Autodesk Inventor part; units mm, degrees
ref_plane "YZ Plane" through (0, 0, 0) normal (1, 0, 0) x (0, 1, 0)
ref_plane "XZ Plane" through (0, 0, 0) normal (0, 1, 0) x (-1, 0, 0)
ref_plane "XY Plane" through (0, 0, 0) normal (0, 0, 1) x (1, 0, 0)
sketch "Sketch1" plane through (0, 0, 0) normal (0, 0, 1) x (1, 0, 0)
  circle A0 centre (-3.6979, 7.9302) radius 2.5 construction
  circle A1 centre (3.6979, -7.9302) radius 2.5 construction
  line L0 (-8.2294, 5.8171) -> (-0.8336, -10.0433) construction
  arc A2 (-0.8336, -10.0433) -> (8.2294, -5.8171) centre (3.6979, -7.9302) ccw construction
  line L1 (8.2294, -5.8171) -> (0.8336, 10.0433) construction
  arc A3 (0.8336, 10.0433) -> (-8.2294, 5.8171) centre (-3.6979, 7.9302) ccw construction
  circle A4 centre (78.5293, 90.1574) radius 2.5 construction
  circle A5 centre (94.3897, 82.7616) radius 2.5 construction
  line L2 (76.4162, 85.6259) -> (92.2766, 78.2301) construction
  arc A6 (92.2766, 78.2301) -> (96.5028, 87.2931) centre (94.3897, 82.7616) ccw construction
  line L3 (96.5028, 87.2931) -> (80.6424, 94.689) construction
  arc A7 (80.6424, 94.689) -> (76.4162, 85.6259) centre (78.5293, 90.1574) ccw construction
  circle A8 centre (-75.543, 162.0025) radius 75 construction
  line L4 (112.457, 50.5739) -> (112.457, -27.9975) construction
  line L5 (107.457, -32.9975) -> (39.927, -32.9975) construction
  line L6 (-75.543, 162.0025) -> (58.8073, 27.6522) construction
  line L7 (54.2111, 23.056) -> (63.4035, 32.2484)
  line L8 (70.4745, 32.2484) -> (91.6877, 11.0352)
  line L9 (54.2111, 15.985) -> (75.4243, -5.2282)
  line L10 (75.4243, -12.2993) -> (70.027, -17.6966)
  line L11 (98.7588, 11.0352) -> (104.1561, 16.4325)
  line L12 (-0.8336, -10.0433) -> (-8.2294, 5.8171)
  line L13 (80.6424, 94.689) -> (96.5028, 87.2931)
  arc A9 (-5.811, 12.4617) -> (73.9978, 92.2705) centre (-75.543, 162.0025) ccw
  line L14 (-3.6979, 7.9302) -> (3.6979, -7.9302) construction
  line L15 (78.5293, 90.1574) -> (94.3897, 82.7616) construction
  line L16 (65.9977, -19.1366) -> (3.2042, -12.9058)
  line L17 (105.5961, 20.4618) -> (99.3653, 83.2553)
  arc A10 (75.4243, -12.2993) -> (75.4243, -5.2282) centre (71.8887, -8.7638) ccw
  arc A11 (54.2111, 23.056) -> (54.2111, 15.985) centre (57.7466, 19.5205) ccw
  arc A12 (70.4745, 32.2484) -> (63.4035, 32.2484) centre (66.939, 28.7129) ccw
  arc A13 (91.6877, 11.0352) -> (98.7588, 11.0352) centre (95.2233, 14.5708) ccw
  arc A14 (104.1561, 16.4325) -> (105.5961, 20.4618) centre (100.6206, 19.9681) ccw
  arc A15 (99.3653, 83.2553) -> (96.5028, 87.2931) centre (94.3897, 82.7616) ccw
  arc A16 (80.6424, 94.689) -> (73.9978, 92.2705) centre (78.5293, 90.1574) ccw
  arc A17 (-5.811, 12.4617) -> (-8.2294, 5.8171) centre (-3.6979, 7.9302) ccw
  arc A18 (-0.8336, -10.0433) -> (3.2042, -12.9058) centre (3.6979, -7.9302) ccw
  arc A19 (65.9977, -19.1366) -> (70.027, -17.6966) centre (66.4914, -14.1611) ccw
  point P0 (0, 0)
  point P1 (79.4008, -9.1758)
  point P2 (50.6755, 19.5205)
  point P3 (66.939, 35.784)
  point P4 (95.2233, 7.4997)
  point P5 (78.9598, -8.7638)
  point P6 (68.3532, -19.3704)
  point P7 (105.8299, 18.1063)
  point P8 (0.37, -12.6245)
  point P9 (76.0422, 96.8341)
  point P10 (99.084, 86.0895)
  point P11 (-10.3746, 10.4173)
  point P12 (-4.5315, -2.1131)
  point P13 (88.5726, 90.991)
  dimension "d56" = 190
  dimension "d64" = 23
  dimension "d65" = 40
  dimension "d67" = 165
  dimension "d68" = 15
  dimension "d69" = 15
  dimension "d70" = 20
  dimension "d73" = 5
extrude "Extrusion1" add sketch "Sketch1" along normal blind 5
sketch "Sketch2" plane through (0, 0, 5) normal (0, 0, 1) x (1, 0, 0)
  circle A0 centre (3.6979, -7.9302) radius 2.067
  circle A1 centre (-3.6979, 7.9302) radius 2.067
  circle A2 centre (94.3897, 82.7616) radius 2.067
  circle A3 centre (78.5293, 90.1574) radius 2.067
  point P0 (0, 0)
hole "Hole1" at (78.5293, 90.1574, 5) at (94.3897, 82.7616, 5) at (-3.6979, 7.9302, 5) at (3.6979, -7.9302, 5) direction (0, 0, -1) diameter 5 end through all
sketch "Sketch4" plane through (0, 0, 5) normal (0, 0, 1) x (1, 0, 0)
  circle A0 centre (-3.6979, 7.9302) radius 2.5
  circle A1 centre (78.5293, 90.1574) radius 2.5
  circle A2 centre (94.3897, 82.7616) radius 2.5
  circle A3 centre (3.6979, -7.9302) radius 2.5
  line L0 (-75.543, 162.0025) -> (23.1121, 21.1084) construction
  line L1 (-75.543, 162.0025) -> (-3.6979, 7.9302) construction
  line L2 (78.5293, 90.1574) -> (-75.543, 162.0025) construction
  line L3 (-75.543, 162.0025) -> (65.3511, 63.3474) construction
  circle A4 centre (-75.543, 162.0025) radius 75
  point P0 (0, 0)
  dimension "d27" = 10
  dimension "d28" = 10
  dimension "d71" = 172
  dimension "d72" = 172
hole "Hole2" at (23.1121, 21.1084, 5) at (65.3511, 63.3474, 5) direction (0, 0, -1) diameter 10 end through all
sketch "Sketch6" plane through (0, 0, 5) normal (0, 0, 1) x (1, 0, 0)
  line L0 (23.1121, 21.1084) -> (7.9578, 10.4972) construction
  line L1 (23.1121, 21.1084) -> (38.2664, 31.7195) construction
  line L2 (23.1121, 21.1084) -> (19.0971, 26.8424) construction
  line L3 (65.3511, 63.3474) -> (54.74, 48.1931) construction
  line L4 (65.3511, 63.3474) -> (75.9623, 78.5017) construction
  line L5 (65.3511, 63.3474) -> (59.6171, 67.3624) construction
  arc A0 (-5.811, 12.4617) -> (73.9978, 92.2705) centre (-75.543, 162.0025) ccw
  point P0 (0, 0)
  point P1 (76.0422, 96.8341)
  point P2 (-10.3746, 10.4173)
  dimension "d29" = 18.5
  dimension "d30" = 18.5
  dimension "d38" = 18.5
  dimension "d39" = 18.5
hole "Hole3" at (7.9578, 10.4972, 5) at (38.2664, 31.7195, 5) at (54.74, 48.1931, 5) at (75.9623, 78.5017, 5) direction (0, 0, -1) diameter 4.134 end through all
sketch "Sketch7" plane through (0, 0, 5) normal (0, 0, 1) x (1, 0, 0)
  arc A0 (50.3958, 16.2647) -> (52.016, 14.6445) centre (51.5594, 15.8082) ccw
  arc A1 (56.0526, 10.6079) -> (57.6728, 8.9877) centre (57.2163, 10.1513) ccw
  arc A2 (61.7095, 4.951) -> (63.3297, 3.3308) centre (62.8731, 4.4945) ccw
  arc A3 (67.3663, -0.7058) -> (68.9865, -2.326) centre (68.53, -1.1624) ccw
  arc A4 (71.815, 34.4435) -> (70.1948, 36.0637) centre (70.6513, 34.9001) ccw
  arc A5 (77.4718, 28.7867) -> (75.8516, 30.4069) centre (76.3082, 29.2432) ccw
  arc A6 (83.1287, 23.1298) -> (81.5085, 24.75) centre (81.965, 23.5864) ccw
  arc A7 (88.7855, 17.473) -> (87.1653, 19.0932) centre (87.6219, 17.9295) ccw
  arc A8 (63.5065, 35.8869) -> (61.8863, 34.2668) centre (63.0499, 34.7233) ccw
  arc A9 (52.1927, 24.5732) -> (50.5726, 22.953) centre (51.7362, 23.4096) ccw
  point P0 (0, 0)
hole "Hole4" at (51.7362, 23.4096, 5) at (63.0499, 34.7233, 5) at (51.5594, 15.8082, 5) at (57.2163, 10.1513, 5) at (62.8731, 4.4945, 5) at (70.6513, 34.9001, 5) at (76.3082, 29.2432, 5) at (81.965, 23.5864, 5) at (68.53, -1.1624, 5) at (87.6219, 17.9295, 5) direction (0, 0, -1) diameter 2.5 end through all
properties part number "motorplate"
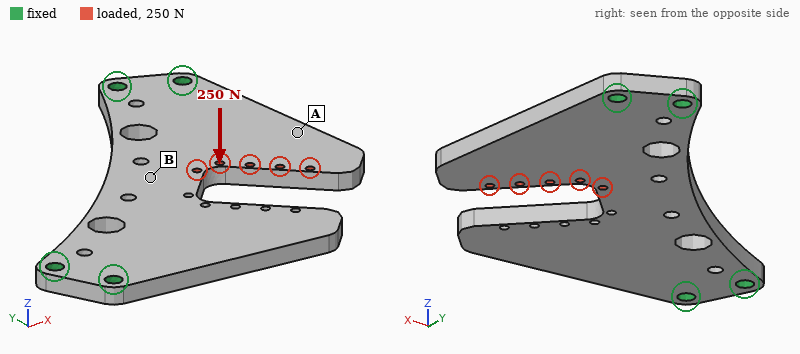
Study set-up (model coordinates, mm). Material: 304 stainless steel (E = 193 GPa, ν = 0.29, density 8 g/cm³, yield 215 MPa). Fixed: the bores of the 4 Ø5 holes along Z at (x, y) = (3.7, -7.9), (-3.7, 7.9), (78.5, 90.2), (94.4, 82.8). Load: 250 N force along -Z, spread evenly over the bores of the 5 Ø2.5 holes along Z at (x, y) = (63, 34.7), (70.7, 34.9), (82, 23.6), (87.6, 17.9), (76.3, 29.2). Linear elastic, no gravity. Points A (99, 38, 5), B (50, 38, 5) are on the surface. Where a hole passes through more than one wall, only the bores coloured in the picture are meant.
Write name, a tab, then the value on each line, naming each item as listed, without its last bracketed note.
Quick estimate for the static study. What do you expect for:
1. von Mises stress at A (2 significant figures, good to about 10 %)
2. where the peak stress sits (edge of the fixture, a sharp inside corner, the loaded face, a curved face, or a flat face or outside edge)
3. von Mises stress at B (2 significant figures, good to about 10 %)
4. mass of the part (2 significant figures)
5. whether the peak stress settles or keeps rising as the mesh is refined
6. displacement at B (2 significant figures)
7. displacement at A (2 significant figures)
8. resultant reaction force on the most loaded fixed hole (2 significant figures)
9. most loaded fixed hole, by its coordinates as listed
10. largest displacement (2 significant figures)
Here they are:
von Mises stress at A	11 MPa
where the peak stress sits	edge of the fixture
von Mises stress at B	27 MPa
mass of the part	240 g
whether the peak stress settles or keeps rising as the mesh is refined	keeps rising
displacement at B	0.043 mm
displacement at A	0.078 mm
resultant reaction force on the most loaded fixed hole	250 N
most loaded fixed hole, by its coordinates as listed	(94.4, 82.8)
largest displacement	0.16 mm
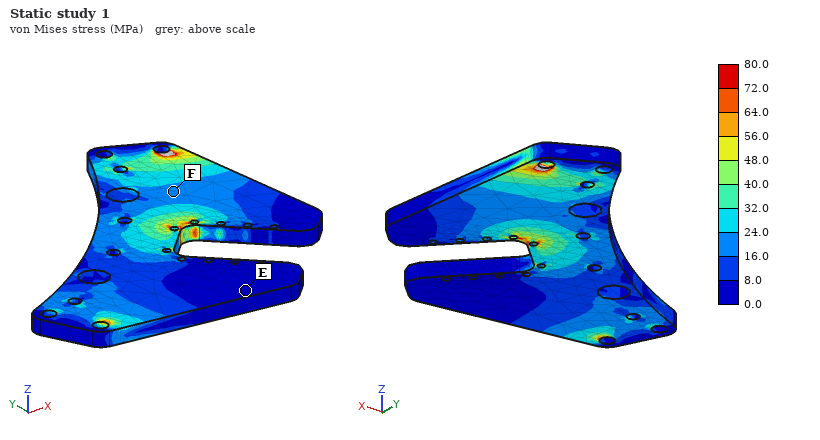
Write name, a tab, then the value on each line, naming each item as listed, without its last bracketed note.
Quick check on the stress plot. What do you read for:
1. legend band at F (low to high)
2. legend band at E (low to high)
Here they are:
legend band at F	16.0 to 24.0 MPa
legend band at E	0.0 to 8.0 MPa
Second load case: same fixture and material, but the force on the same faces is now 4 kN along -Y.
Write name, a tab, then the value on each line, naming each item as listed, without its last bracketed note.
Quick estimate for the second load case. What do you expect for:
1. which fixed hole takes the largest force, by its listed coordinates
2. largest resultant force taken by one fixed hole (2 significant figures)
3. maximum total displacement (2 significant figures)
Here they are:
which fixed hole takes the largest force, by its listed coordinates	(78.5, 90.2)
largest resultant force taken by one fixed hole	2.4 kN
maximum total displacement	19 µm
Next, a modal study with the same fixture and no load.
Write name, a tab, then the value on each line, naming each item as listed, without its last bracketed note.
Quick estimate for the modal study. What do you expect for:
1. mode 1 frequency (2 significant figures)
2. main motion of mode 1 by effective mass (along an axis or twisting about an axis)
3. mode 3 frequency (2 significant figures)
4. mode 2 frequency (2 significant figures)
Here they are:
mode 1 frequency	910 Hz
main motion of mode 1 by effective mass	along Z
mode 3 frequency	2200 Hz
mode 2 frequency	1500 Hz
